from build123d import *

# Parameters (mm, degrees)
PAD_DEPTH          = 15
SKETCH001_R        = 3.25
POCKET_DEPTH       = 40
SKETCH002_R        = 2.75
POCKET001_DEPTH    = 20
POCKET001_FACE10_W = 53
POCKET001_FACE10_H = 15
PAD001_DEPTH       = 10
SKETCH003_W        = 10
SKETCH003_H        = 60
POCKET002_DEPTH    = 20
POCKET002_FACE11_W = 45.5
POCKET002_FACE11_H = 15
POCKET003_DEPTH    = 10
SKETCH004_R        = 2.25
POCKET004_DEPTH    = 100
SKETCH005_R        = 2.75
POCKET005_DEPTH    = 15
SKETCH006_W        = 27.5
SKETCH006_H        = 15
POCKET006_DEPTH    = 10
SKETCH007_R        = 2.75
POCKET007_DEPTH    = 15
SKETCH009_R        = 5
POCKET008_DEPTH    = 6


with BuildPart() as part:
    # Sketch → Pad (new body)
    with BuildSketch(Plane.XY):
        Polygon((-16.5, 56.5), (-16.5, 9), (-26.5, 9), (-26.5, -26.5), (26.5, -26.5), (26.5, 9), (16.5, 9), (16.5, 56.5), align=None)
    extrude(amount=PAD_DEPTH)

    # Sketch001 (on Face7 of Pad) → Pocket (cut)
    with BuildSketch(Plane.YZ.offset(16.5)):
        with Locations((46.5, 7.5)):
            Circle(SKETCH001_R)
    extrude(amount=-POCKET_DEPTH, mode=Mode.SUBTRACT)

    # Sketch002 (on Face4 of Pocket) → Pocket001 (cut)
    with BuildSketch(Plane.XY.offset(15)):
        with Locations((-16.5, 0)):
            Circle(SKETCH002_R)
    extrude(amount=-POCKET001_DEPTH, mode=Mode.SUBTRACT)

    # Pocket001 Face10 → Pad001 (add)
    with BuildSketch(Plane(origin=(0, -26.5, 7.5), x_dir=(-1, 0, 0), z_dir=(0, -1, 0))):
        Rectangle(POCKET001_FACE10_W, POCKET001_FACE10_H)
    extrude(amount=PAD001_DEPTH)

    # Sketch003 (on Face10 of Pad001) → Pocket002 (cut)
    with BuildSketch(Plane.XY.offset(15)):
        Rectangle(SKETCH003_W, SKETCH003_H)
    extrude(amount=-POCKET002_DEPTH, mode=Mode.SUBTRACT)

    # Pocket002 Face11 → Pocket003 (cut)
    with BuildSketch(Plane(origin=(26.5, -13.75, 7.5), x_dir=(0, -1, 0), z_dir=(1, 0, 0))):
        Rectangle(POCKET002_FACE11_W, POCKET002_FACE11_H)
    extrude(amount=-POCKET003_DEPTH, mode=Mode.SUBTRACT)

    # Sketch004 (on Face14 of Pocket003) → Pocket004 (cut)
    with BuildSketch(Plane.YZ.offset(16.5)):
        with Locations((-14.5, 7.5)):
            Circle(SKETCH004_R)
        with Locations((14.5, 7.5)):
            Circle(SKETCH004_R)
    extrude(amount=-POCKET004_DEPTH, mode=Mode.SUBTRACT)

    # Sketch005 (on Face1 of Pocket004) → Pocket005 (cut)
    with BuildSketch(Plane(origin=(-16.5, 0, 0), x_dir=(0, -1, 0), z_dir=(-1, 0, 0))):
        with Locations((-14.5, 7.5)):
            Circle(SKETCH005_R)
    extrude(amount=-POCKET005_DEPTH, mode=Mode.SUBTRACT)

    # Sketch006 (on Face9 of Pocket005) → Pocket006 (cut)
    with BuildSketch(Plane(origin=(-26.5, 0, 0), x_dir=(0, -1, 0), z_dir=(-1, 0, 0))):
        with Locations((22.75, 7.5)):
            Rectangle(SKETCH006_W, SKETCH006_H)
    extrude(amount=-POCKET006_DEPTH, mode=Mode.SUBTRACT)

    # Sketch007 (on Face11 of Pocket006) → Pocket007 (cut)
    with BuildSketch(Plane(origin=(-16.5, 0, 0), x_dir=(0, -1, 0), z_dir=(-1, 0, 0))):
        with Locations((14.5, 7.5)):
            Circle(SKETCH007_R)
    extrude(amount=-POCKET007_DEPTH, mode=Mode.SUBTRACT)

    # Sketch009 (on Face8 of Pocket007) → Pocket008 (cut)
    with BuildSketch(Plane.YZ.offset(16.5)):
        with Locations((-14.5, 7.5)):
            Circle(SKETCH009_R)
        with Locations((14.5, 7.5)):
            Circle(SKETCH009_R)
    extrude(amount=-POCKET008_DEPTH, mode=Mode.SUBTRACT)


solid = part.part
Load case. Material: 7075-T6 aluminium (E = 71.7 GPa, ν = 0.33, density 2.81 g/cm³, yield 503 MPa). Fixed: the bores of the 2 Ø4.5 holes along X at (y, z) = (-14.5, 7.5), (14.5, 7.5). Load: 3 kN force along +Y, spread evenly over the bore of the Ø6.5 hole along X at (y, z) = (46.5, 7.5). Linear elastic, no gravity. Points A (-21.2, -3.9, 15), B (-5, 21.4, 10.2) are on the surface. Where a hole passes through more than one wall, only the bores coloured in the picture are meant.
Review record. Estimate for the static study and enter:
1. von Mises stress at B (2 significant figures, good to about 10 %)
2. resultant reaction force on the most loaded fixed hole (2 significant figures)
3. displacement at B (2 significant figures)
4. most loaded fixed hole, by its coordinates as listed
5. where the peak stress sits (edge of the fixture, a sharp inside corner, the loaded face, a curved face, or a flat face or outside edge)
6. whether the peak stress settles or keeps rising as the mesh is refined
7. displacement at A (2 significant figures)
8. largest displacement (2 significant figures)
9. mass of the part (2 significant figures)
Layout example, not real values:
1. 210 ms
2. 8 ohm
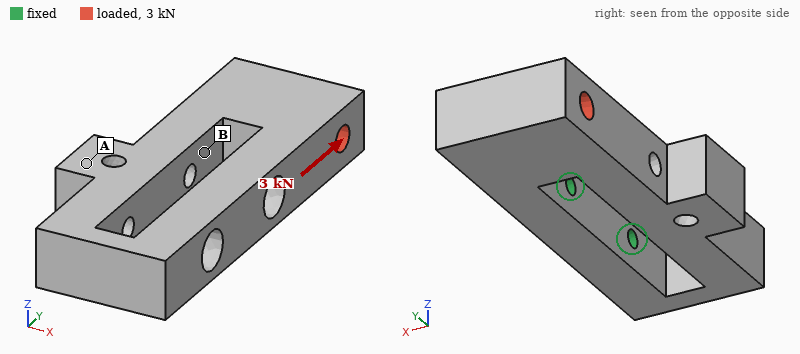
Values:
1. 14 MPa
2. 2.2 kN
3. 39 µm
4. (14.5, 7.5)
5. edge of the fixture
6. keeps rising
7. 47 µm
8. 90 µm
9. 100 g
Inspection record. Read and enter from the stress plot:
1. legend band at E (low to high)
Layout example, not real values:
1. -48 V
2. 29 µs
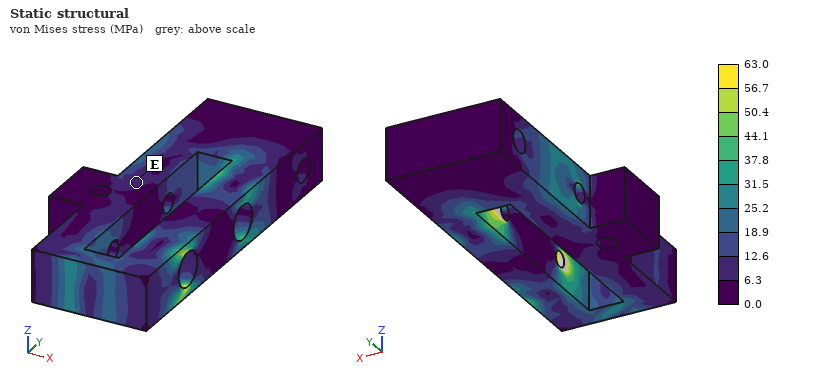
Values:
1. 6.3 to 12.6 MPa
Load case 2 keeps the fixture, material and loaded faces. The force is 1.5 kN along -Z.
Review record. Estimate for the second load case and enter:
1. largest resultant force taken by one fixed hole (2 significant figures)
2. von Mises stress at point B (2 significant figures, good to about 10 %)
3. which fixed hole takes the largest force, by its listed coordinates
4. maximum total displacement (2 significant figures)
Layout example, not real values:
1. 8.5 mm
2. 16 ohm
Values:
1. 2.7 kN
2. 19 MPa
3. (14.5, 7.5)
4. 0.23 mm
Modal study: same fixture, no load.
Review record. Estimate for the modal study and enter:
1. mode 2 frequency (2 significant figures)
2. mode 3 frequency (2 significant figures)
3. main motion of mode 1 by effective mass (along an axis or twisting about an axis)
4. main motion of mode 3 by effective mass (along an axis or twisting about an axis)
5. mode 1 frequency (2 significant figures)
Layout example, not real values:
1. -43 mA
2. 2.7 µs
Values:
1. 2700 Hz
2. 3400 Hz
3. along Z
4. twisting about X
5. 2200 Hz
